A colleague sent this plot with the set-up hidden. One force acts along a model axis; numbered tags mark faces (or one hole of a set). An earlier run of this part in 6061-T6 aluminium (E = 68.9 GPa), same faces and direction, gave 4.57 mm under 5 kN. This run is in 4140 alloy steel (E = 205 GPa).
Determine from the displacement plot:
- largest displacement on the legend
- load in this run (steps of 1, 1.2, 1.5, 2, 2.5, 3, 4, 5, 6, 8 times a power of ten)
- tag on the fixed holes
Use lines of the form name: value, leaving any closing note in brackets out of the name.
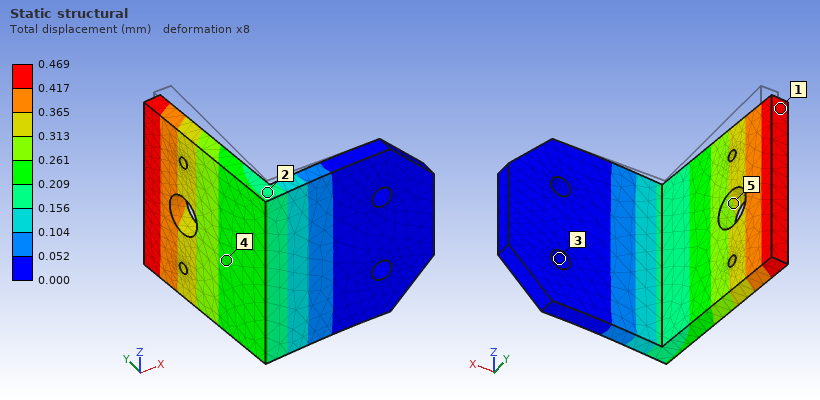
largest displacement on the legend: 0.469 mm
load in this run: 1.5 kN
tag on the fixed holes: 3
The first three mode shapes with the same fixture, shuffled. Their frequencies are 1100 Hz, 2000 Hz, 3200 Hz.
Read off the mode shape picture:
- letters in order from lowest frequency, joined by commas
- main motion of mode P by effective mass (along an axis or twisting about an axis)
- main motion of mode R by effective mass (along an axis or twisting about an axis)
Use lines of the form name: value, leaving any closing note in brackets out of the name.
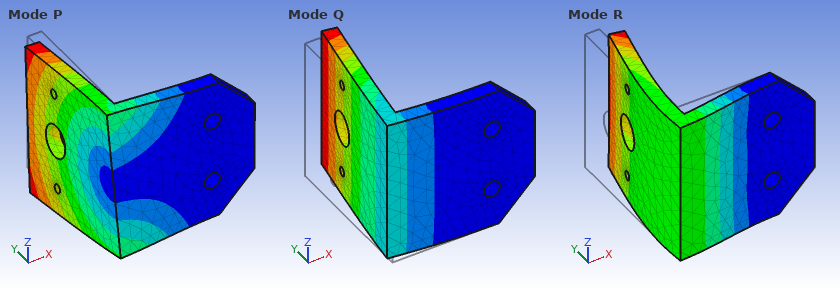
letters in order from lowest frequency, joined by commas: Q, P, R
main motion of mode P by effective mass: along Z
main motion of mode R by effective mass: along Y
